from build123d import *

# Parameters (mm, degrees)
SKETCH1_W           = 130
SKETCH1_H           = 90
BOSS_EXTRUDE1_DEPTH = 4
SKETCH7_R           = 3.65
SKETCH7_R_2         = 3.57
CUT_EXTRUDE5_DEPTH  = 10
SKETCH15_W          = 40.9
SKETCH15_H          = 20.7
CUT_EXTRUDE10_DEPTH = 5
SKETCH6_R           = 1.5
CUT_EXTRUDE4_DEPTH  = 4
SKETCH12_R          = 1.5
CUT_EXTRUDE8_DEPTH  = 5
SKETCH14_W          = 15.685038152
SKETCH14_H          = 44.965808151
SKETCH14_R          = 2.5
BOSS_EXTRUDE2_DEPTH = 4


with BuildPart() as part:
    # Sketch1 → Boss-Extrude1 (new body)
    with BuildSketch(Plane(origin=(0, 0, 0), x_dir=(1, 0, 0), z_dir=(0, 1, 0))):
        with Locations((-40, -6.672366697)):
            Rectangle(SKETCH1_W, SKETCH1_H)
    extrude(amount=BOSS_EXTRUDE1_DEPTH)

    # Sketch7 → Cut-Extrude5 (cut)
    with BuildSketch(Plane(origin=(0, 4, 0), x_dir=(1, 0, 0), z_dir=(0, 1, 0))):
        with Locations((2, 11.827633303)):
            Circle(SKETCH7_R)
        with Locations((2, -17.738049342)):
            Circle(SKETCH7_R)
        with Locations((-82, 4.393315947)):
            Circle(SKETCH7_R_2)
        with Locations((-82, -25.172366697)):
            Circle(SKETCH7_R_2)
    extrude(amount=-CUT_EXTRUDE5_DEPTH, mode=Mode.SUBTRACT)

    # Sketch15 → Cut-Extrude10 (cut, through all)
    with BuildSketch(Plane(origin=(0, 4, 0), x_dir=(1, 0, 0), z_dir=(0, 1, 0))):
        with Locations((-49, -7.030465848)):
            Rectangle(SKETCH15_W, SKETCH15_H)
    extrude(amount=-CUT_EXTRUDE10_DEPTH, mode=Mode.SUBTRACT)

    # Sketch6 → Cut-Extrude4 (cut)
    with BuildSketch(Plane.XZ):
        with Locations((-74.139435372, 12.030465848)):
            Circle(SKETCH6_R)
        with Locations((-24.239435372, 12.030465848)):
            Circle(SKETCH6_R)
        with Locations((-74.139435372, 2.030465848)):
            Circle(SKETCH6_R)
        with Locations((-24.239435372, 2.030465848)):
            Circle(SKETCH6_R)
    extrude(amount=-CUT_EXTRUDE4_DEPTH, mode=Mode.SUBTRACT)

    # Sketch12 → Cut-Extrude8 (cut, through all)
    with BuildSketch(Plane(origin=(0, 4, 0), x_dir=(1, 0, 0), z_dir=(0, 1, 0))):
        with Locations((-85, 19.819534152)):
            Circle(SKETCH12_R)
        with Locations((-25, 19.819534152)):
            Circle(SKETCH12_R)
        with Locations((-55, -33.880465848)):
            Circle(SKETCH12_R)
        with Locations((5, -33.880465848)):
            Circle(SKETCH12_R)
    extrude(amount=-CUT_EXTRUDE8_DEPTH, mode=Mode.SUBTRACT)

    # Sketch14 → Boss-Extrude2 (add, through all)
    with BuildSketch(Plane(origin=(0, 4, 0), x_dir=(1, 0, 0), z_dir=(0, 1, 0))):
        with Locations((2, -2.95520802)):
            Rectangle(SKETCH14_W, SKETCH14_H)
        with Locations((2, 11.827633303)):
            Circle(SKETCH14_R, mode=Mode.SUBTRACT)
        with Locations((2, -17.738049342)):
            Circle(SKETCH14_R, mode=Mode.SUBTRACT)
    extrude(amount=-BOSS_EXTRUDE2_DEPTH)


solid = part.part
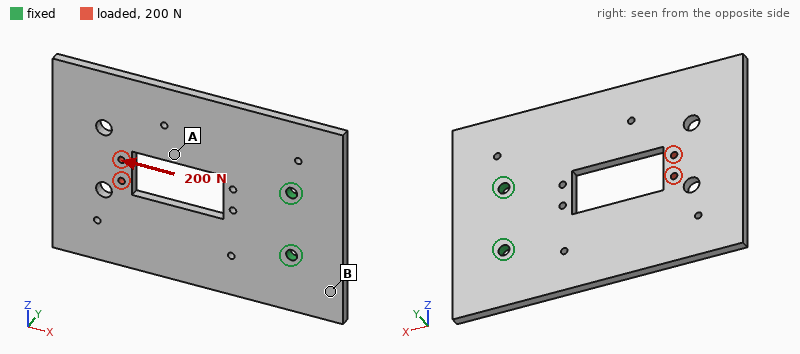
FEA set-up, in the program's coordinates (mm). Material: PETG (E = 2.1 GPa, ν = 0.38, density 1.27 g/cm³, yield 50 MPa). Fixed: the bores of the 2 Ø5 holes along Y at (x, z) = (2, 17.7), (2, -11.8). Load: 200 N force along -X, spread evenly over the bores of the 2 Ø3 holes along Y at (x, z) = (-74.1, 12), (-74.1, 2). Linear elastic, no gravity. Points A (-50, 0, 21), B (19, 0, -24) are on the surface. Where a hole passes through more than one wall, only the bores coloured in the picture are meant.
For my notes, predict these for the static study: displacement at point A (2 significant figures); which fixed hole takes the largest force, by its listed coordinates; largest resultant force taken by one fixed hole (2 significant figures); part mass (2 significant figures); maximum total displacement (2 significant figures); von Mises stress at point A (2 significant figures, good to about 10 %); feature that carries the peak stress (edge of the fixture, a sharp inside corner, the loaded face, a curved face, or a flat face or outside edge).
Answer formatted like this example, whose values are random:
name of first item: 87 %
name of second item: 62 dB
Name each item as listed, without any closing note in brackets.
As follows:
displacement at point A: 43 µm
which fixed hole takes the largest force, by its listed coordinates: (2, 17.7)
largest resultant force taken by one fixed hole: 120 N
part mass: 54 g
maximum total displacement: 79 µm
von Mises stress at point A: 1.5 MPa
feature that carries the peak stress: the loaded face
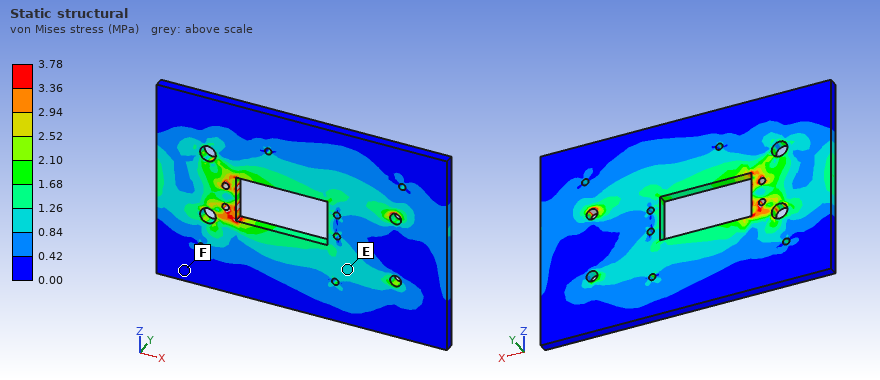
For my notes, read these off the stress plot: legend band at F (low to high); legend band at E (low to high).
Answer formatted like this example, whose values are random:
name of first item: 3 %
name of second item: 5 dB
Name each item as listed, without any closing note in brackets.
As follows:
legend band at F: 0.00 to 0.42 MPa
legend band at E: 0.84 to 1.26 MPa
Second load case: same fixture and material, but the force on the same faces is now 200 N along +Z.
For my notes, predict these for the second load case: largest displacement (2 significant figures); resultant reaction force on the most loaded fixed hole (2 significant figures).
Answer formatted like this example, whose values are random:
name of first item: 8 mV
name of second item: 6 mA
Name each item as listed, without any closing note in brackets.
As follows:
largest displacement: 0.63 mm
resultant reaction force on the most loaded fixed hole: 480 N
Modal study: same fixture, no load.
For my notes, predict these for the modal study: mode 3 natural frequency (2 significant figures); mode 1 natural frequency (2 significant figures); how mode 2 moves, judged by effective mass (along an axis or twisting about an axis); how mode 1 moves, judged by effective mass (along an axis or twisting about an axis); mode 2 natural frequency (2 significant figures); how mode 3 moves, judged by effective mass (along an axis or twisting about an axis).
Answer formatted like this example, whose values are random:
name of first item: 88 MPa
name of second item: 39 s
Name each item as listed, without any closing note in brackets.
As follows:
mode 3 natural frequency: 400 Hz
mode 1 natural frequency: 69 Hz
how mode 2 moves, judged by effective mass: twisting about X
how mode 1 moves, judged by effective mass: along Y
mode 2 natural frequency: 170 Hz
how mode 3 moves, judged by effective mass: along Y
